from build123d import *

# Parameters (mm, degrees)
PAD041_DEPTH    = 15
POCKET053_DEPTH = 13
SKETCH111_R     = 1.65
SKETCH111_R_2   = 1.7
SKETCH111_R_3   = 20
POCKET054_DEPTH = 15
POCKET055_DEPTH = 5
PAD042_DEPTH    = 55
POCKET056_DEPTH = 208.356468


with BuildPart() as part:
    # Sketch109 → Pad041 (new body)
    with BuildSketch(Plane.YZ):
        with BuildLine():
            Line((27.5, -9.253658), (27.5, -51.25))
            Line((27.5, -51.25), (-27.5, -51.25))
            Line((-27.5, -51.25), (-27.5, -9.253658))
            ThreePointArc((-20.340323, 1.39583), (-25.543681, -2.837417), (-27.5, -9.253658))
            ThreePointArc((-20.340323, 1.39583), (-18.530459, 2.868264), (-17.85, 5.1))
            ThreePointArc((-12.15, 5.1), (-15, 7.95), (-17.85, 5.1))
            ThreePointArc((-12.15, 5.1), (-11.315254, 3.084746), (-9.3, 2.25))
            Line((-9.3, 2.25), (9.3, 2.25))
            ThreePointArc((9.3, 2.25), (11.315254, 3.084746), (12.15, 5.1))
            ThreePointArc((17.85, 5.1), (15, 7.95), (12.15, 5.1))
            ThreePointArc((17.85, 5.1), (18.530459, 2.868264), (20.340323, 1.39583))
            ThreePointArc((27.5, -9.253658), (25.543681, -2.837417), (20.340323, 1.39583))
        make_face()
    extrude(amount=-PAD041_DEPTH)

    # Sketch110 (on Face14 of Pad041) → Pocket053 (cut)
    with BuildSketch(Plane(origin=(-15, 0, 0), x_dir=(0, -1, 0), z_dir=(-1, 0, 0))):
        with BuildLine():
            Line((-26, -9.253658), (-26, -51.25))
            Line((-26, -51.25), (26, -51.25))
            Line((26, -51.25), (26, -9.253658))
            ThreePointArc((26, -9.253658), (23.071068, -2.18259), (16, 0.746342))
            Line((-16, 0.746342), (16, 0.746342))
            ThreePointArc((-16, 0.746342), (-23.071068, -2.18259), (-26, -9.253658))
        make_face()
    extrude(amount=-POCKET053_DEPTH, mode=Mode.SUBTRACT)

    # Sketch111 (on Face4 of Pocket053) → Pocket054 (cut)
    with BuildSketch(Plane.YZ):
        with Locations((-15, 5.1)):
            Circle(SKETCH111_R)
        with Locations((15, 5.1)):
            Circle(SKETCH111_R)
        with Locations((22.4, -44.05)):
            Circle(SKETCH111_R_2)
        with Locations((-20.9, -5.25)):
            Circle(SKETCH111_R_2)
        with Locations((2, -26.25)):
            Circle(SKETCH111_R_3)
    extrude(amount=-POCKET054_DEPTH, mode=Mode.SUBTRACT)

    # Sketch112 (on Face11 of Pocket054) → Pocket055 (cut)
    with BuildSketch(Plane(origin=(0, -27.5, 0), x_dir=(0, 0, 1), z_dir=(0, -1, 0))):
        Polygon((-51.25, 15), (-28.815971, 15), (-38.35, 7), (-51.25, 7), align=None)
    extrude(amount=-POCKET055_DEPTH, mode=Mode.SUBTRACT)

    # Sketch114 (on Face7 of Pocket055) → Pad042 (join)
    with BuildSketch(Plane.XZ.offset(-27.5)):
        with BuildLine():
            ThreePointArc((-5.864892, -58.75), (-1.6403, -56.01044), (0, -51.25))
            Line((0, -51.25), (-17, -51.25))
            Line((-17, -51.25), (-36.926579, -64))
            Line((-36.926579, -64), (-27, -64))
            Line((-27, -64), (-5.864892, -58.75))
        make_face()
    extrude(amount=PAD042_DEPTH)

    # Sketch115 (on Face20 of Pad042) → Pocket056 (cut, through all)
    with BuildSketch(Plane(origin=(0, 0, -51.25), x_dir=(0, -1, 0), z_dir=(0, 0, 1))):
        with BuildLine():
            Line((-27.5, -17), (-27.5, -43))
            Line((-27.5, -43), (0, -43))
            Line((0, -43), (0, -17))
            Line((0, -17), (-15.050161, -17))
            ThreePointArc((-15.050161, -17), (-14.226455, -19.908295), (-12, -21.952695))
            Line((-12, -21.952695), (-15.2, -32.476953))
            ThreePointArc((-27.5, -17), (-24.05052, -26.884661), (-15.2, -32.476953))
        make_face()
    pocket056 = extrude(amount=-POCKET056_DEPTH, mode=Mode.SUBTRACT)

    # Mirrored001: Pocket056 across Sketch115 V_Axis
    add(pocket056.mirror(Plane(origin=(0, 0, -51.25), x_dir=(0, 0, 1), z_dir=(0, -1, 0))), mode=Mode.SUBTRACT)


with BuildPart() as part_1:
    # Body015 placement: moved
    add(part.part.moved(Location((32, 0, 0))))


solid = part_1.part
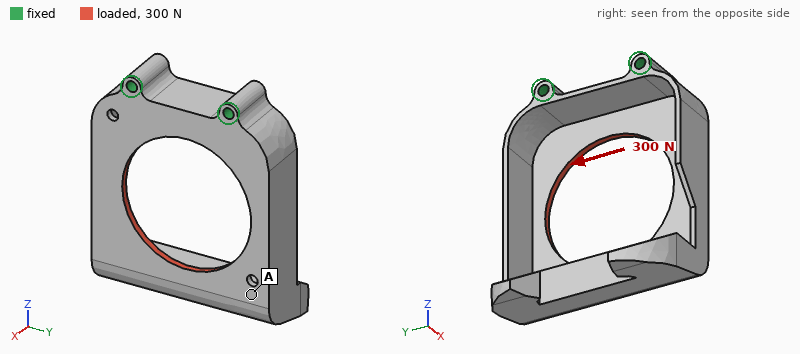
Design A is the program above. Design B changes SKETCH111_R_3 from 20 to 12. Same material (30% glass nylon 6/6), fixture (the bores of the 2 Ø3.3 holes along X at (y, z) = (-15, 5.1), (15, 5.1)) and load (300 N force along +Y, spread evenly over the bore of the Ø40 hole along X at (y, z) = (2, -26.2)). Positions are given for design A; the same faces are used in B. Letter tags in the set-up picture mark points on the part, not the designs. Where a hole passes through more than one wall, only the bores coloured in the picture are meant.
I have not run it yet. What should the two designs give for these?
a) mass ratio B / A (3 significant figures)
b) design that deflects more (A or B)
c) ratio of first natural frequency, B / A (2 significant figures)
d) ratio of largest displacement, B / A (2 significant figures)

1.10
A
1.0
0.35
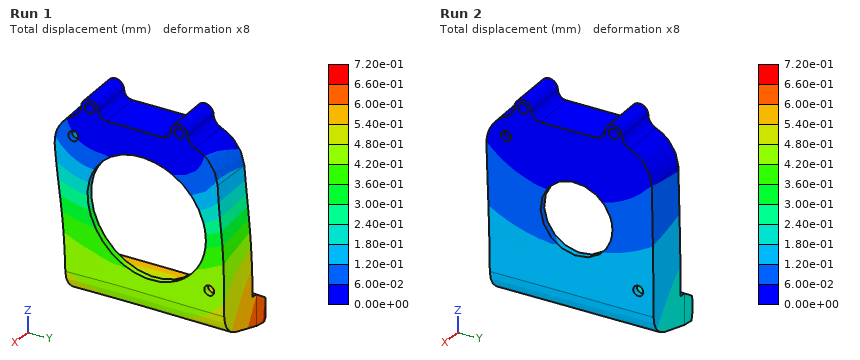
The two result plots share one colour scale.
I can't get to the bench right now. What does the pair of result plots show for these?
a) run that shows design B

Run 2
